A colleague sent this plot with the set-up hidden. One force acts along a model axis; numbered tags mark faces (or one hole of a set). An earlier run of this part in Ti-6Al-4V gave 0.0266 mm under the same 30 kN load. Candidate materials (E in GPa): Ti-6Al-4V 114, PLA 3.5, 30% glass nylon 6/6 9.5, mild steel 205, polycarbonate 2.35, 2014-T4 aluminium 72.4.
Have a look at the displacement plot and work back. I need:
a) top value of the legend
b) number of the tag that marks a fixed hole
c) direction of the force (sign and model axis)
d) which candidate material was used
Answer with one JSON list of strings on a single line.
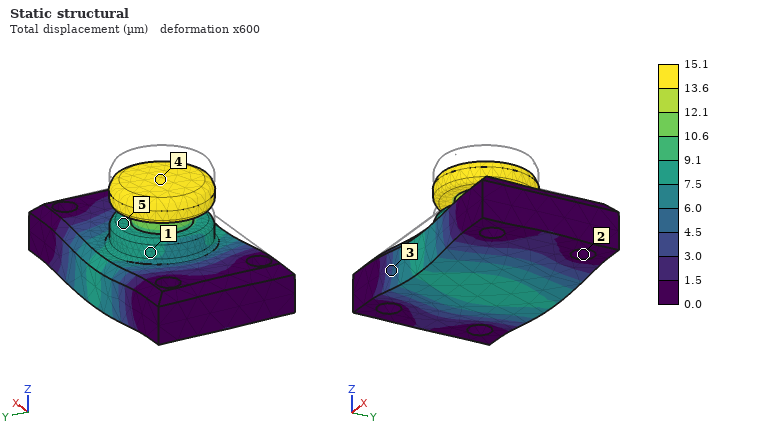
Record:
["15.1 µm", "2", "-Z", "mild steel"]
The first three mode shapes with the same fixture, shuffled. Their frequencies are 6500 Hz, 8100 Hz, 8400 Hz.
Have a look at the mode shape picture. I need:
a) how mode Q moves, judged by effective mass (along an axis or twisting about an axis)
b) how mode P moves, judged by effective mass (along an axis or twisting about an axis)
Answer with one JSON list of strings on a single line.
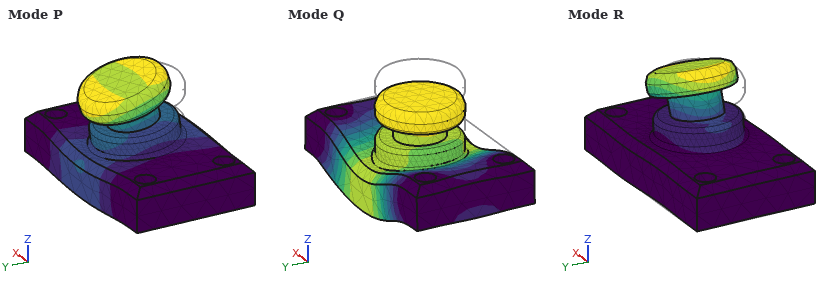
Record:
["along Z", "along Y"]
